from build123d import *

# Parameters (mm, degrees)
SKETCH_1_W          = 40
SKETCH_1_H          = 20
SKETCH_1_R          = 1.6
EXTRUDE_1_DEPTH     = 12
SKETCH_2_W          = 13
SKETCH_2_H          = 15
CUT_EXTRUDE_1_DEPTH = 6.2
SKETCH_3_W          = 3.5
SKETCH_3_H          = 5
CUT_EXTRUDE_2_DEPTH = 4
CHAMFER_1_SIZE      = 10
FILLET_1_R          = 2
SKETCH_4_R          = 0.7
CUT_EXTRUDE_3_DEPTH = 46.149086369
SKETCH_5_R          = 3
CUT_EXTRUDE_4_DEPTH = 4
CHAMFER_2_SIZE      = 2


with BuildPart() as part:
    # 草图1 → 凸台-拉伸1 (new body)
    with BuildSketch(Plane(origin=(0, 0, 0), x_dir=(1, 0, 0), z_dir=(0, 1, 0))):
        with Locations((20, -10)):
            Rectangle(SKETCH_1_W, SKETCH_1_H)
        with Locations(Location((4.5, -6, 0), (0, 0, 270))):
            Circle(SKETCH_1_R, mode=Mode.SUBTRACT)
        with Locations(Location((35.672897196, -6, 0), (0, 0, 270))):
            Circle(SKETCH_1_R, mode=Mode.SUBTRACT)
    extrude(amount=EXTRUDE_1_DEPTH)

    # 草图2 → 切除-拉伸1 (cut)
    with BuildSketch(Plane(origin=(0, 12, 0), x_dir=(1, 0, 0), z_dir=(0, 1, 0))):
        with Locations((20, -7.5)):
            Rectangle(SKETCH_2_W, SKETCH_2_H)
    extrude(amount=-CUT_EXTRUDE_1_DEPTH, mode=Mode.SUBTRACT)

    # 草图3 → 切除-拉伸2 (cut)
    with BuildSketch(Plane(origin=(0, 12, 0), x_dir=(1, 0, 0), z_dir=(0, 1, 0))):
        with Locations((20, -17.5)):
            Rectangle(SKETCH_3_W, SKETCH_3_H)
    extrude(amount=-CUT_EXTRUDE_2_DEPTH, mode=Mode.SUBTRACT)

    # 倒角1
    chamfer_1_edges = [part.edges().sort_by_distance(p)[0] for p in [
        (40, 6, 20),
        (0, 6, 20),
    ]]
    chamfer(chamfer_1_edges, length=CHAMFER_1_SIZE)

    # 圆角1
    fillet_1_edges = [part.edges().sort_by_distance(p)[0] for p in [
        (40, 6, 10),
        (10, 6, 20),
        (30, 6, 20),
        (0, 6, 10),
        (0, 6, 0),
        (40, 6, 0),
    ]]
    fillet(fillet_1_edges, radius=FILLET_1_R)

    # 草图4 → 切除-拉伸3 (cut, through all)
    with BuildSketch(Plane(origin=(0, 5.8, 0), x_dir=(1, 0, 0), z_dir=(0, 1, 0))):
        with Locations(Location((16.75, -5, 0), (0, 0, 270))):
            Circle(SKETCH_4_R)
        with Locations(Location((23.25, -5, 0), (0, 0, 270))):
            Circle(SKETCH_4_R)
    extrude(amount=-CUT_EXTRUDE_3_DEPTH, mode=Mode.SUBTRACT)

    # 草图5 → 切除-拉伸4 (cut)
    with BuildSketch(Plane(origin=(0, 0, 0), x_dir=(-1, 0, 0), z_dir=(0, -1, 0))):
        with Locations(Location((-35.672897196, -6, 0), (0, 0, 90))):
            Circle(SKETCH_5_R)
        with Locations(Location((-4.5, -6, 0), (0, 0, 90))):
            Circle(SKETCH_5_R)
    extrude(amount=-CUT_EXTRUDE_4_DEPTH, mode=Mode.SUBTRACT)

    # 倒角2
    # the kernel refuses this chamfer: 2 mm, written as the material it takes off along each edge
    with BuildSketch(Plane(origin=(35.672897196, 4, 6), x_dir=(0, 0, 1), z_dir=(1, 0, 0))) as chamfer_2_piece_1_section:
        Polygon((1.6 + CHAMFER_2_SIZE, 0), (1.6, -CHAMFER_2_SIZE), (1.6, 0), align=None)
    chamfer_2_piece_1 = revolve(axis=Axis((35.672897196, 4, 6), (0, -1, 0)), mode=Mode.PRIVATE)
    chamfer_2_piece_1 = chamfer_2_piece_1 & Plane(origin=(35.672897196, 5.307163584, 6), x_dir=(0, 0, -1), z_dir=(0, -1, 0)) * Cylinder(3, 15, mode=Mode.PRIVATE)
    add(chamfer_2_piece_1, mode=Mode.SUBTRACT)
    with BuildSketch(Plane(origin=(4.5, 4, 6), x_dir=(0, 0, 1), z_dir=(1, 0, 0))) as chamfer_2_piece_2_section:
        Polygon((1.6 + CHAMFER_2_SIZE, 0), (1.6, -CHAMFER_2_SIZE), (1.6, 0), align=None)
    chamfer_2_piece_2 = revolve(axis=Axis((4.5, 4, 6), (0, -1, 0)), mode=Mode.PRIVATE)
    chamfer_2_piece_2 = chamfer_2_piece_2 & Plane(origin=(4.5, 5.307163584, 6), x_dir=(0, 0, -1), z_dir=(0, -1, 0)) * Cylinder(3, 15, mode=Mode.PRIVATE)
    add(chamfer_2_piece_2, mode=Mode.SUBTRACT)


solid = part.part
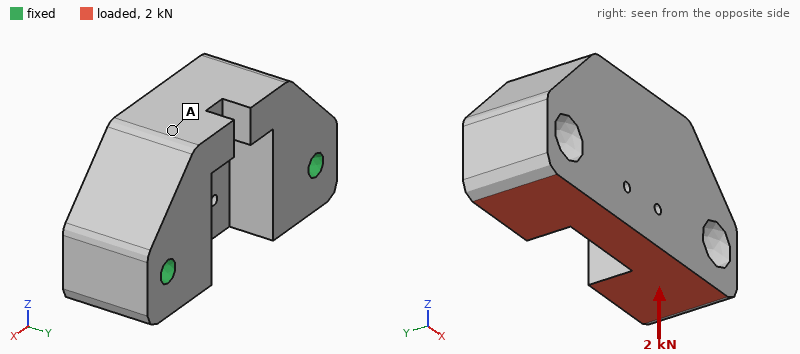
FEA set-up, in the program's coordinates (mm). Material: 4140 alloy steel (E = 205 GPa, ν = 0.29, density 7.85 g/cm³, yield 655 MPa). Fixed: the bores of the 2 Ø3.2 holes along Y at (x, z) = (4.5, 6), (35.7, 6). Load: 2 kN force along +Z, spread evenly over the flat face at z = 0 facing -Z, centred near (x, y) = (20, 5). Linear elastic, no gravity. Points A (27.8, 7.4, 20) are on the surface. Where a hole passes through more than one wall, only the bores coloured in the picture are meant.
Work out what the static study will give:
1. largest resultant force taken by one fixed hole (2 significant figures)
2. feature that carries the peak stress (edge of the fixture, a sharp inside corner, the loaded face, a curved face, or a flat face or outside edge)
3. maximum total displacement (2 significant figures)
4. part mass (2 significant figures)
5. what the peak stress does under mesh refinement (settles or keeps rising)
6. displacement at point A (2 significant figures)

1.0 kN
edge of the fixture
3.6 µm
52 g
keeps rising
2.6 µm
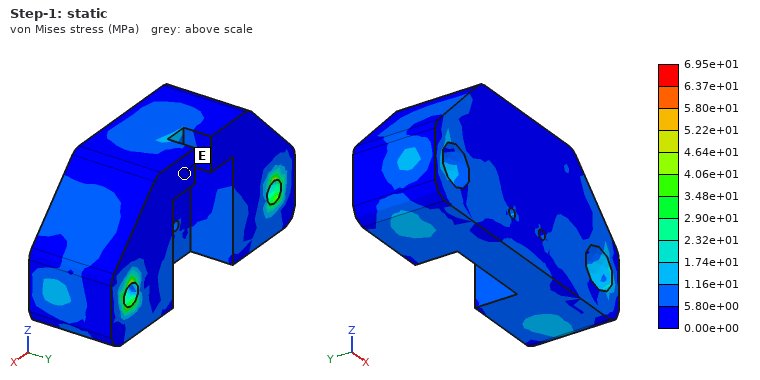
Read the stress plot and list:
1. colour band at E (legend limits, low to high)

0.00e+00 to 5.80e+00 MPa
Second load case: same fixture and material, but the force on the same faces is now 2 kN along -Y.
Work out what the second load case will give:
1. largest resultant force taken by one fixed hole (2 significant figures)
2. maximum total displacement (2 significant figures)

1.1 kN
5.6 µm
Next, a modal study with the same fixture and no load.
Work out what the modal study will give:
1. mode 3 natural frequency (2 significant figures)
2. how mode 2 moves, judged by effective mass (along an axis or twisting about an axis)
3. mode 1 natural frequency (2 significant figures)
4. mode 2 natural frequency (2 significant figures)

32 kHz
along X
15 kHz
30 kHz
